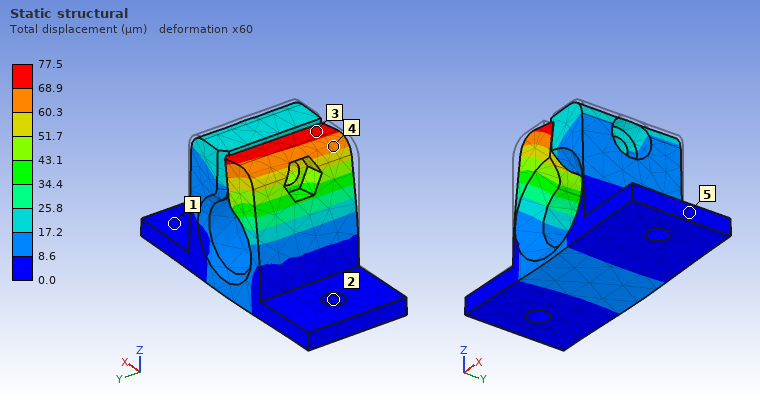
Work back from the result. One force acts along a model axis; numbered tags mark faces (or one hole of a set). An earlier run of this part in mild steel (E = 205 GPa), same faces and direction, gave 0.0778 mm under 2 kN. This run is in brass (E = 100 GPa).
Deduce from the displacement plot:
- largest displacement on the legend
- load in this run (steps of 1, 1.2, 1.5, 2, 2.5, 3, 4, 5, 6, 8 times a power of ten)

77.5 µm
1 kN
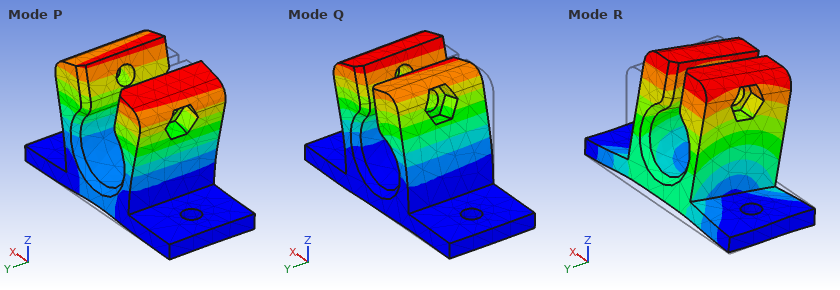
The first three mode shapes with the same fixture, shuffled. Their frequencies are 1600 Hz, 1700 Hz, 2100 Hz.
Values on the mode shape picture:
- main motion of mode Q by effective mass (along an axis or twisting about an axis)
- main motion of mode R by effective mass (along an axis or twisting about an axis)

along X
along Y
